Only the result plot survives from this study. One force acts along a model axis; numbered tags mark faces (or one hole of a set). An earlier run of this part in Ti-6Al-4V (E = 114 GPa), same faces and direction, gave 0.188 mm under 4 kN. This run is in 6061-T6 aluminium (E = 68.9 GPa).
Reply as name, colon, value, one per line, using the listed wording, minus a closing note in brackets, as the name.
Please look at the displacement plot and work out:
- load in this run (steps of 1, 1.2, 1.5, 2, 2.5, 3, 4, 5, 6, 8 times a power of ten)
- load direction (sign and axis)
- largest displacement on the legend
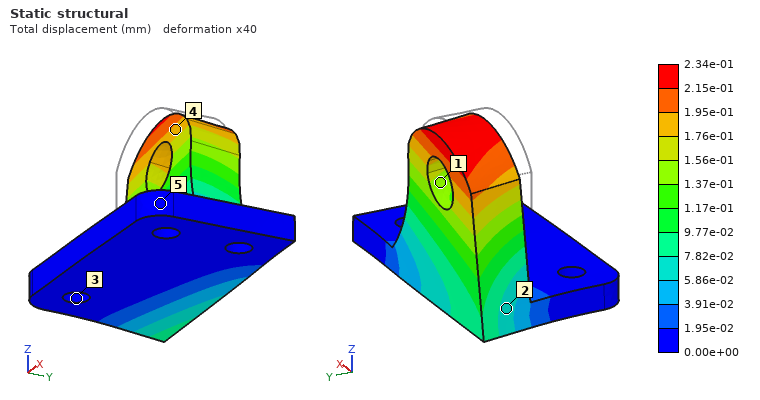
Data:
load in this run: 3 kN
load direction: +Y
largest displacement on the legend: 2.34e-01 mm
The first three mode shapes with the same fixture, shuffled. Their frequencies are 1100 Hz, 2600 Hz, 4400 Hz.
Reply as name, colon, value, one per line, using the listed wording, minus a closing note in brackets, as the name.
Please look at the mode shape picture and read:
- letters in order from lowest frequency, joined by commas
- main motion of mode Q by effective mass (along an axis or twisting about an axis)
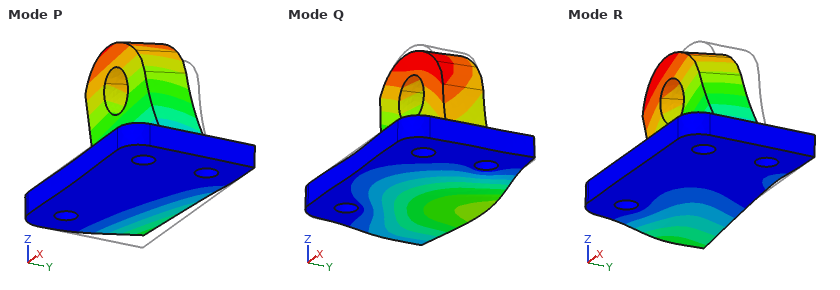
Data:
letters in order from lowest frequency, joined by commas: P, R, Q
main motion of mode Q by effective mass: along Z
